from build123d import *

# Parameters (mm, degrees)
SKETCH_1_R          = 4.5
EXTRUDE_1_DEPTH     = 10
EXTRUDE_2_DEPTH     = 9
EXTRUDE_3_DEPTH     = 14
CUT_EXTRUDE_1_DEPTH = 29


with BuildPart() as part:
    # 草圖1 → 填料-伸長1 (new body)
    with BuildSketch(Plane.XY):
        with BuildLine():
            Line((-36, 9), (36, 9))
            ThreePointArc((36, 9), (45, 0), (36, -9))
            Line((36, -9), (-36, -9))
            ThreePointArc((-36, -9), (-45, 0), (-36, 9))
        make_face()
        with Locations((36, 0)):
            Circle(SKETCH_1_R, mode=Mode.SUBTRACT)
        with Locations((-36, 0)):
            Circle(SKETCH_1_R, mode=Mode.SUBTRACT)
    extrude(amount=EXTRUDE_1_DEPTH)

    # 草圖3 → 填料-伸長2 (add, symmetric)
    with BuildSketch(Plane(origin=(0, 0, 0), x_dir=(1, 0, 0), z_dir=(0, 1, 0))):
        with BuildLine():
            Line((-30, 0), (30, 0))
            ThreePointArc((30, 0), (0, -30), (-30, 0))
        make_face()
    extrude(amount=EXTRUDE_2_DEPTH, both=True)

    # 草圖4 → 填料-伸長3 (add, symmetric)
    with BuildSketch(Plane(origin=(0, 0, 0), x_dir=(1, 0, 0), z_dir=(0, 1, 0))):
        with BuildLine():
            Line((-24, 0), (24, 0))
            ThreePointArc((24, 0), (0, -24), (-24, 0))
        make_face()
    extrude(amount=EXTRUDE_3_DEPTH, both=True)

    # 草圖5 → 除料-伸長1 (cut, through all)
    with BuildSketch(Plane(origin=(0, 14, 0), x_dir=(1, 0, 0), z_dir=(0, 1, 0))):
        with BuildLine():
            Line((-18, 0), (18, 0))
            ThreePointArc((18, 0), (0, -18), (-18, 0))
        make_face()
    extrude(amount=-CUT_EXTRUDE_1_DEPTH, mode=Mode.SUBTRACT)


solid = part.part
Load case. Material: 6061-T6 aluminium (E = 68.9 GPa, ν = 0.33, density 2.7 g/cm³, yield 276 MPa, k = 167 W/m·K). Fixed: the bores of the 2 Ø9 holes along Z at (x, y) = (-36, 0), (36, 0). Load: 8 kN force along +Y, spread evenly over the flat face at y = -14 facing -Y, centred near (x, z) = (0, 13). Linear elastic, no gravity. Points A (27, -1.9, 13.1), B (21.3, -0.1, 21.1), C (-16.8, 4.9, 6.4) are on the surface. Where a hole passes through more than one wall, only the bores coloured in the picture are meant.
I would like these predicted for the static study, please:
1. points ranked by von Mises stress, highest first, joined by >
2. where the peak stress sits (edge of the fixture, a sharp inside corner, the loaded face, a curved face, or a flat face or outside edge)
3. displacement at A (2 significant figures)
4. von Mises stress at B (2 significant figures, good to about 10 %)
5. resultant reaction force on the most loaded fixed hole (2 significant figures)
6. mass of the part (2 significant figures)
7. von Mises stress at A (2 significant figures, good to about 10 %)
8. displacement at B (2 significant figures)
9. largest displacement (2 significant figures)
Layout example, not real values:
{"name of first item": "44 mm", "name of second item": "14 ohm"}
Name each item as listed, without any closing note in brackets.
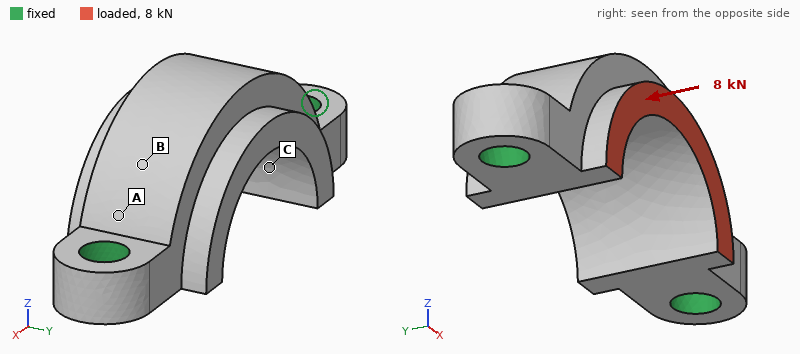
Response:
{"points ranked by von Mises stress, highest first, joined by >": "A > B > C", "where the peak stress sits": "edge of the fixture", "displacement at A": "0.032 mm", "von Mises stress at B": "44 MPa", "resultant reaction force on the most loaded fixed hole": "4.0 kN", "mass of the part": "64 g", "von Mises stress at A": "73 MPa", "displacement at B": "0.066 mm", "largest displacement": "0.11 mm"}
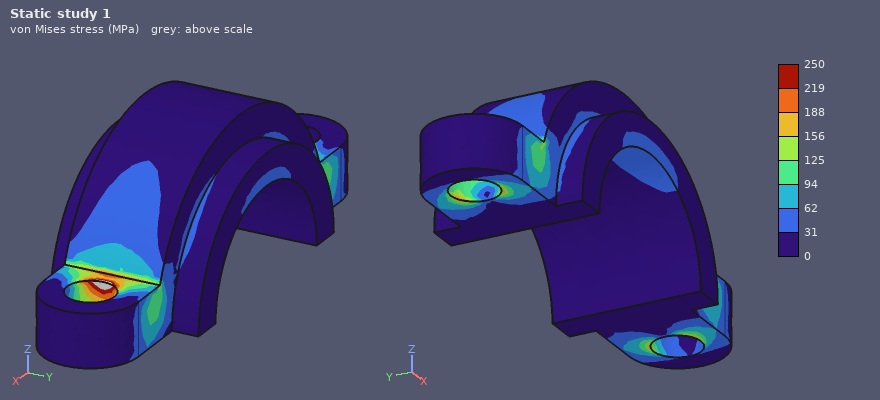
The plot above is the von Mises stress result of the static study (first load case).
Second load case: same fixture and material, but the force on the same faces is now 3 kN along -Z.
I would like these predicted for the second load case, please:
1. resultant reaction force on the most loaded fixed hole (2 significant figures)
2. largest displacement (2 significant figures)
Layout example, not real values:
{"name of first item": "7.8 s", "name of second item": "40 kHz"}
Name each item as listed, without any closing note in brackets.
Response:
{"resultant reaction force on the most loaded fixed hole": "1.9 kN", "largest displacement": "55 µm"}
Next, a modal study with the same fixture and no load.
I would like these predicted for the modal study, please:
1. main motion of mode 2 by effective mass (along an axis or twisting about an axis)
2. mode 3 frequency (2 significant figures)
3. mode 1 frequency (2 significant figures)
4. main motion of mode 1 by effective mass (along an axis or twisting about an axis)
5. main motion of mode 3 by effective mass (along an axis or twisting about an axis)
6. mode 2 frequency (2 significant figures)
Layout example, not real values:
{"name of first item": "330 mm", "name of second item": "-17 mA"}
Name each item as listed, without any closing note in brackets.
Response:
{"main motion of mode 2 by effective mass": "along Z", "mode 3 frequency": "16 kHz", "mode 1 frequency": "6500 Hz", "main motion of mode 1 by effective mass": "along Y", "main motion of mode 3 by effective mass": "along X", "mode 2 frequency": "15 kHz"}
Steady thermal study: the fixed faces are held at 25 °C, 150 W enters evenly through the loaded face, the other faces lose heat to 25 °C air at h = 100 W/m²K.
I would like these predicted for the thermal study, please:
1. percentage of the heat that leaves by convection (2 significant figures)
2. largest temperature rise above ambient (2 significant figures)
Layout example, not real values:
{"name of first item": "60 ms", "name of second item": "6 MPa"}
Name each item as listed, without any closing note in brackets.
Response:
{"percentage of the heat that leaves by convection": "12 %", "largest temperature rise above ambient": "57 K"}
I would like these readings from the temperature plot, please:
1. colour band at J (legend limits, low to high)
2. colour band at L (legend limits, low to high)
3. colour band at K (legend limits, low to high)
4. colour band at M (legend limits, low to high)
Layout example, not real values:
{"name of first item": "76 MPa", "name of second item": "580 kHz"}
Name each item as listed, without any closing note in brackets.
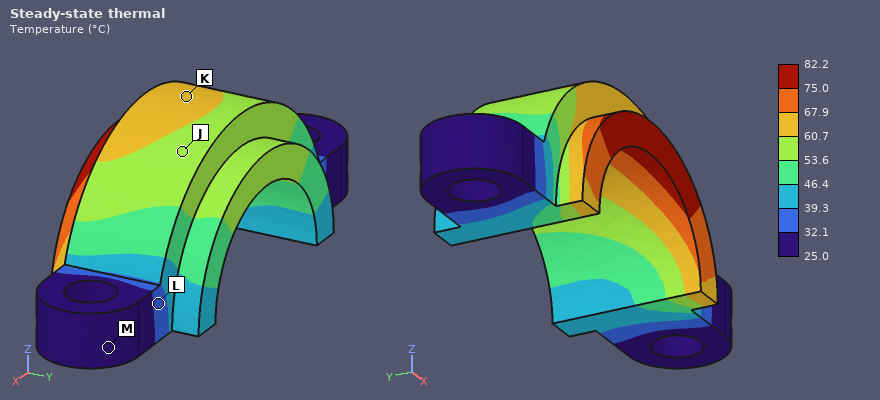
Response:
{"colour band at J": "53.6 to 60.7 °C", "colour band at L": "32.1 to 39.3 °C", "colour band at K": "60.7 to 67.9 °C", "colour band at M": "25.0 to 32.1 °C"}
